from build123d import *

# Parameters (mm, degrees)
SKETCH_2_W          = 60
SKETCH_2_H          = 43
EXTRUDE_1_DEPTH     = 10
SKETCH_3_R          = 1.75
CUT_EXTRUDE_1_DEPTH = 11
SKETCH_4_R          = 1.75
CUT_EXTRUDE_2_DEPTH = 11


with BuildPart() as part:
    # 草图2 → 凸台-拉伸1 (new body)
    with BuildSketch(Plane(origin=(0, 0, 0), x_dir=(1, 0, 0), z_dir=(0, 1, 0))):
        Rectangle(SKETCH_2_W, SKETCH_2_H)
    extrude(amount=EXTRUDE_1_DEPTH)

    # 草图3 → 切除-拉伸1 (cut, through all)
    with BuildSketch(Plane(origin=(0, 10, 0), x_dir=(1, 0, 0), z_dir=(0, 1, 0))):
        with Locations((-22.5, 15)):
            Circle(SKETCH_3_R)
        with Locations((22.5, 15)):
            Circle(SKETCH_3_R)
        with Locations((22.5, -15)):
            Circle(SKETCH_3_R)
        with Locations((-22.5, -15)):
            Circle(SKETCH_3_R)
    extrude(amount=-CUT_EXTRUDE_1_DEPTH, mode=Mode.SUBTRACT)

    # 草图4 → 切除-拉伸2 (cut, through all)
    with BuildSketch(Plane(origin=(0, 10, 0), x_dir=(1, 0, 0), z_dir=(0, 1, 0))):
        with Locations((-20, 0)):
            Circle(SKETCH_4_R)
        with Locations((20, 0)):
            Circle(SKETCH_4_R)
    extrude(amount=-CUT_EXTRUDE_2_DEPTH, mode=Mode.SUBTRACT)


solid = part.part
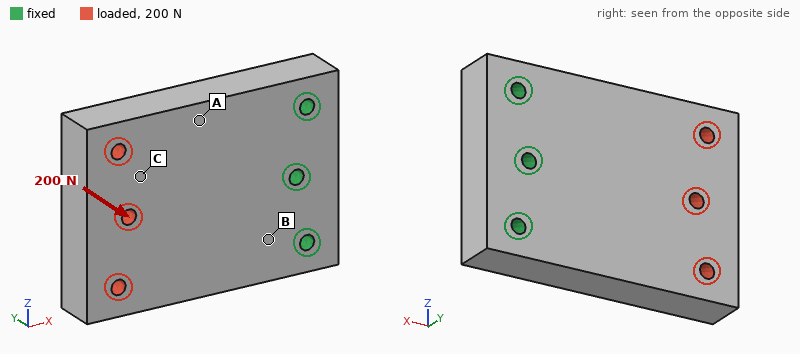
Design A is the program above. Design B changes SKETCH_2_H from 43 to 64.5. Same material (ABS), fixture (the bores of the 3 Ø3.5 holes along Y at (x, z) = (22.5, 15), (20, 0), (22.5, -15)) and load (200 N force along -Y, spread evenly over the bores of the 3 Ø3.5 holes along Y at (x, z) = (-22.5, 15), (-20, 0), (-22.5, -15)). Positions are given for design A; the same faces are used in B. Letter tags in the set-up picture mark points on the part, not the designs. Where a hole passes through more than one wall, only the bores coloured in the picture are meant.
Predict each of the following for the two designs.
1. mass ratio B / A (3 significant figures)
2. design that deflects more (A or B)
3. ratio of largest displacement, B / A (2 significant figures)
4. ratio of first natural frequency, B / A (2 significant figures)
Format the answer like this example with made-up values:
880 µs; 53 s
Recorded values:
1.51; A; 0.77; 0.92
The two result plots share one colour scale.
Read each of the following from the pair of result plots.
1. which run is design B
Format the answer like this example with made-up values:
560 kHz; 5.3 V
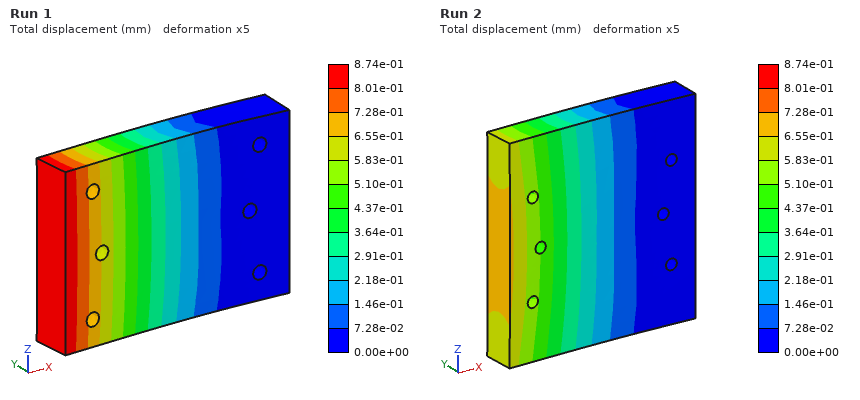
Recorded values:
Run 2
